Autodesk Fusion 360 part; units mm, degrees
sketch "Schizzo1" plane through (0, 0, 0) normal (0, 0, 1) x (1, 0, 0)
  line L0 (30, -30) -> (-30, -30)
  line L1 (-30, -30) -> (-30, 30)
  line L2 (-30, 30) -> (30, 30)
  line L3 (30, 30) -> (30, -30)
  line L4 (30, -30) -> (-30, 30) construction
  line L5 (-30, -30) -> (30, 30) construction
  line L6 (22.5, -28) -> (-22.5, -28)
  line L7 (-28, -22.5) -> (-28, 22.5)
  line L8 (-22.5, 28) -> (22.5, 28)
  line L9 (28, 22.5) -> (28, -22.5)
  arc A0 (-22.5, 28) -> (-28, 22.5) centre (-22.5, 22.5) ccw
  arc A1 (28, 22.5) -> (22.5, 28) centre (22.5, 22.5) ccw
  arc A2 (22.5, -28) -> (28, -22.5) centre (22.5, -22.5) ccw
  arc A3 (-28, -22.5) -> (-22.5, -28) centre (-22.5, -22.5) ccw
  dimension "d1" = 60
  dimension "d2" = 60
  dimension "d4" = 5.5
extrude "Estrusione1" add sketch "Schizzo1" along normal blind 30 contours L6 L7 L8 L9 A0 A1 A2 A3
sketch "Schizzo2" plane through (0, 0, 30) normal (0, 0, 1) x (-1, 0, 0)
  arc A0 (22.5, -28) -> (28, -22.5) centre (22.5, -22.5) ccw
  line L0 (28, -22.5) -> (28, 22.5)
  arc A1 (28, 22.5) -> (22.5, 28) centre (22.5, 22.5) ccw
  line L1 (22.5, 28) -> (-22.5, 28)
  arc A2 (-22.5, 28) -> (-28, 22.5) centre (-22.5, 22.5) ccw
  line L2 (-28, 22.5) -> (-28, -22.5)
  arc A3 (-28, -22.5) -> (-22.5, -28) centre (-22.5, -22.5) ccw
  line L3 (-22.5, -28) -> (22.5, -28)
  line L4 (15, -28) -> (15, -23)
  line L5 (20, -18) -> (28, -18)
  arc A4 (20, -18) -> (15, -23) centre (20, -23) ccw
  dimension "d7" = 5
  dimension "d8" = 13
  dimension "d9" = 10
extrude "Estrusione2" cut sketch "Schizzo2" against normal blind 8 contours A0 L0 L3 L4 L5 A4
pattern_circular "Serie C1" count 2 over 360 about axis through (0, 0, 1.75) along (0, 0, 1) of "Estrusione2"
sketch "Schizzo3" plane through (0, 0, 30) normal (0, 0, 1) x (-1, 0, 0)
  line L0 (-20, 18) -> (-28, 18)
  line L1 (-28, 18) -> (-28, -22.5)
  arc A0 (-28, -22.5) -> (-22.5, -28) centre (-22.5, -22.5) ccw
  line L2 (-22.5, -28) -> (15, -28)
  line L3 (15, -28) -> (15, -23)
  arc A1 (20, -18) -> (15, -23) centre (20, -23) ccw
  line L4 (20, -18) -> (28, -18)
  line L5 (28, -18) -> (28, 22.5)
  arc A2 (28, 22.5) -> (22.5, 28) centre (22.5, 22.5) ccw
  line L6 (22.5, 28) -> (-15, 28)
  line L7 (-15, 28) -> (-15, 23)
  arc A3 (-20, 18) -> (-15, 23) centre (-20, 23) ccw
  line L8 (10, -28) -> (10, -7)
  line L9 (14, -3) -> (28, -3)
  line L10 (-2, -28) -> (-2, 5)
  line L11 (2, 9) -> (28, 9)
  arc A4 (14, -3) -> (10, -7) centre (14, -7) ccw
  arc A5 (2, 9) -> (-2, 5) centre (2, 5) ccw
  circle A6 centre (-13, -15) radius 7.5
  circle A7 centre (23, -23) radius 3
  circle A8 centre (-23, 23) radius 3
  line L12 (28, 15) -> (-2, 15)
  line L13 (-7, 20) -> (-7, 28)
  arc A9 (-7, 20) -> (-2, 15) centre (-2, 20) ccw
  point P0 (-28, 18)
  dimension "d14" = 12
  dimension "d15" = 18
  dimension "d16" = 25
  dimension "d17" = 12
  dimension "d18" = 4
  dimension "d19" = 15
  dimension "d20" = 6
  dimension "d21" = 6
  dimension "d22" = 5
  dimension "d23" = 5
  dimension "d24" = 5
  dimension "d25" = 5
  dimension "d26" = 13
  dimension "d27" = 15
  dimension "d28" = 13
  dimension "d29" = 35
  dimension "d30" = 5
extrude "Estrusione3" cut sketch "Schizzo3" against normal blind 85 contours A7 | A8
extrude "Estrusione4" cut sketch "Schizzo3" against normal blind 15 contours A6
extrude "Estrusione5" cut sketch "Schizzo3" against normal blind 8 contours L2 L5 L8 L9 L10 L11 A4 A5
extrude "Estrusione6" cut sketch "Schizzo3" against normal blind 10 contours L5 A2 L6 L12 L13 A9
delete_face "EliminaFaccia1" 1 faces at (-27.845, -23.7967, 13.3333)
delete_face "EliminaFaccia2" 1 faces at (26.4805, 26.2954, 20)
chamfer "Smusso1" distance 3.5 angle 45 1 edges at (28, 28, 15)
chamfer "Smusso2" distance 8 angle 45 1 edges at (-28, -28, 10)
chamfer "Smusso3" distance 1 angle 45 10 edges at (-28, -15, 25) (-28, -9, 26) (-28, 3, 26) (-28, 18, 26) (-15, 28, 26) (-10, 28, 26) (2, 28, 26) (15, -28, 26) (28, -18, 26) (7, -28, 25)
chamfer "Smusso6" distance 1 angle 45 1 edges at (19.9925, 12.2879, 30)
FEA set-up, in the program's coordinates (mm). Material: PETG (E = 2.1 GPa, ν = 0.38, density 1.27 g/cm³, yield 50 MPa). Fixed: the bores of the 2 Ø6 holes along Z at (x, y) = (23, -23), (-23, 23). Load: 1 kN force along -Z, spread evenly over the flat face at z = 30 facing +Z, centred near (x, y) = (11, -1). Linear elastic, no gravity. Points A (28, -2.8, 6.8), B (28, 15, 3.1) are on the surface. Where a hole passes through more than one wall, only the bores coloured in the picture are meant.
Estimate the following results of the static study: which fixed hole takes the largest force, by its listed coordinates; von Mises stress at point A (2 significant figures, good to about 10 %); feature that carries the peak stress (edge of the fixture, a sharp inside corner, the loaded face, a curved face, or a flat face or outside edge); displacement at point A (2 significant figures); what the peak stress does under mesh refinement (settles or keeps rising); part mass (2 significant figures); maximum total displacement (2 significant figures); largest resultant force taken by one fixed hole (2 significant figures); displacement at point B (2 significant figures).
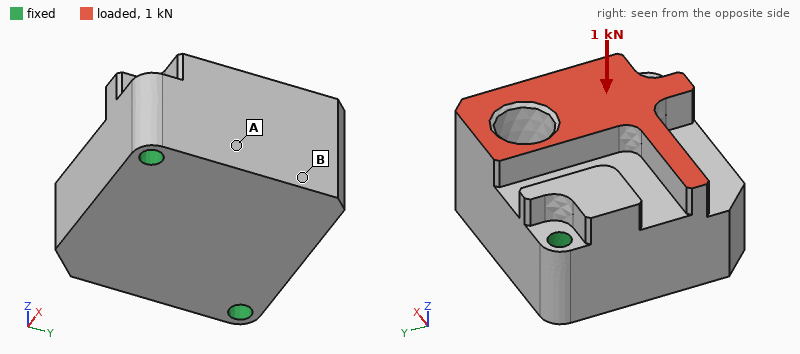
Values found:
(23, -23)
1.9 MPa
edge of the fixture
0.061 mm
keeps rising
98 g
0.15 mm
640 N
0.11 mm
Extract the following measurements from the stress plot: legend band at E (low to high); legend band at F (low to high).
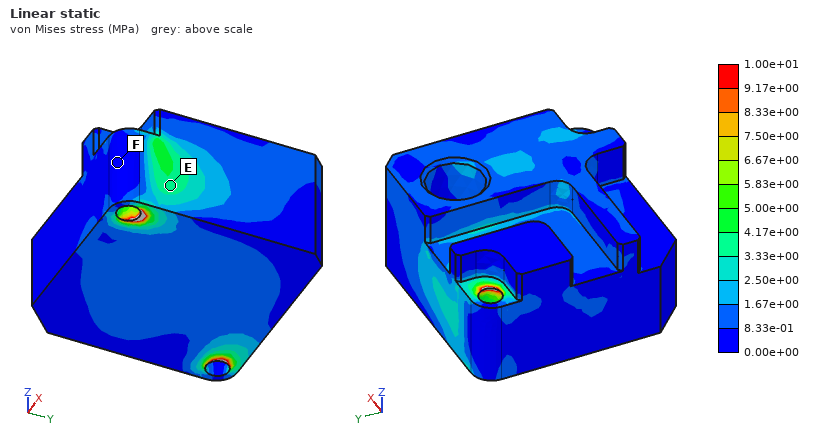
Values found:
3.33e+00 to 4.17e+00 MPa
0.00e+00 to 8.33e-01 MPa
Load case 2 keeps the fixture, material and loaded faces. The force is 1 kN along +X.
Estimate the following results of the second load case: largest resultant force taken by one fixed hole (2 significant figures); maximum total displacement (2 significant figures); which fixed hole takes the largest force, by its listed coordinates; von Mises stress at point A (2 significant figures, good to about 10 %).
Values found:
600 N
0.18 mm
(23, -23)
1.9 MPa
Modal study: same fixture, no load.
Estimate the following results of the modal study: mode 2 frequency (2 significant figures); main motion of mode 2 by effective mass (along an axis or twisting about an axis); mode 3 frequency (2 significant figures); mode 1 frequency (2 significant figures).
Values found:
2600 Hz
along Z
3600 Hz
1900 Hz
